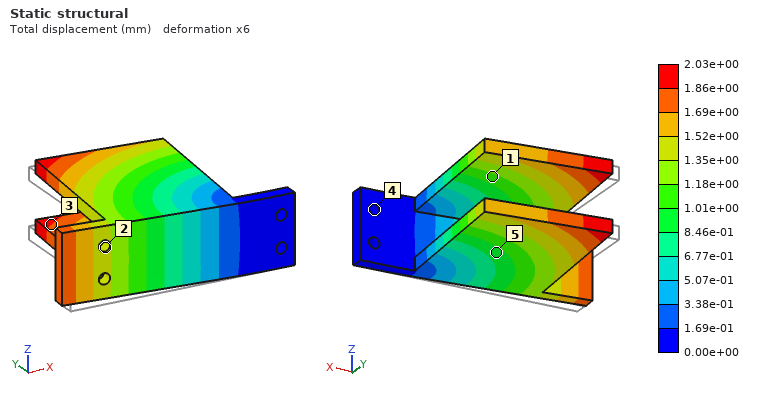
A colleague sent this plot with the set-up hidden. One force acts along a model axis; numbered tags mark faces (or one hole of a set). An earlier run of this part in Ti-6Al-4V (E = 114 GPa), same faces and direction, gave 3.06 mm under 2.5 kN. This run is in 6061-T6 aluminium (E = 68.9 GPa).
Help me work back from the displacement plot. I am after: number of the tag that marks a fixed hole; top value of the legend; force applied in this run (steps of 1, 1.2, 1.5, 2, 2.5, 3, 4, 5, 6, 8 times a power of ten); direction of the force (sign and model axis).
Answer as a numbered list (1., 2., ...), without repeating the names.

1. 4
2. 2.03e+00 mm
3. 1 kN
4. +Y
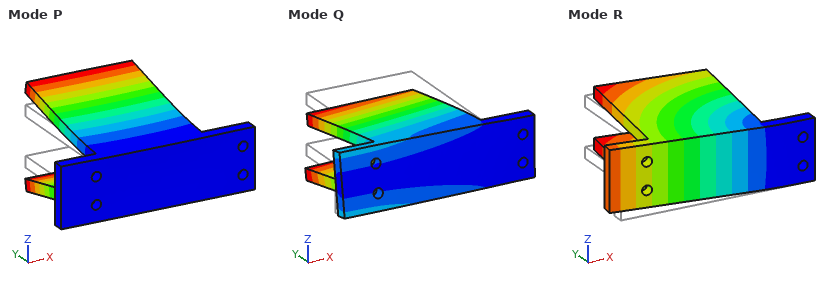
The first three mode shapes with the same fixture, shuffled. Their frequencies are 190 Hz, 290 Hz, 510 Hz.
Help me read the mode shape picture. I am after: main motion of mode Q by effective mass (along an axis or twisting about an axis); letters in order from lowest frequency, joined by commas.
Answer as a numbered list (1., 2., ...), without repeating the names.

1. along Z
2. R, Q, P
